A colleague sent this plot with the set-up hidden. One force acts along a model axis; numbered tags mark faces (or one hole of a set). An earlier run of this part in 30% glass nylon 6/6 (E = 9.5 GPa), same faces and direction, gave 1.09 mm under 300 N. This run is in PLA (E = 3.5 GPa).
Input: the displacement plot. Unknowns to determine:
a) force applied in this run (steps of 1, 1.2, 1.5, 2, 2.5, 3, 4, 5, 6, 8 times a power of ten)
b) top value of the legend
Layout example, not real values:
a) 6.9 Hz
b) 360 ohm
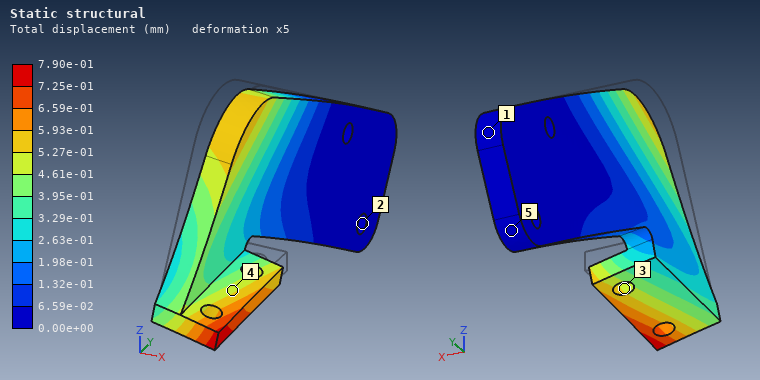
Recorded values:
a) 80 N
b) 7.90e-01 mm
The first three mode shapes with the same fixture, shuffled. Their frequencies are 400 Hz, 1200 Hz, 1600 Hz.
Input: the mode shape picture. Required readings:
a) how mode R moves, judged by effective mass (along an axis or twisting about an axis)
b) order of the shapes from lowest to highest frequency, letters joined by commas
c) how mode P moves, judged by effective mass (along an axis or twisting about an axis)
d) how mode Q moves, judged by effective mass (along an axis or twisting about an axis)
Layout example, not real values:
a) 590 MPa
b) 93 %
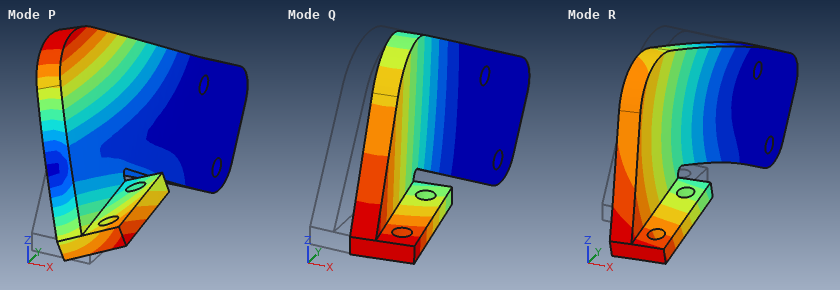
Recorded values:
a) along Z
b) Q, P, R
c) twisting about Y
d) along X
